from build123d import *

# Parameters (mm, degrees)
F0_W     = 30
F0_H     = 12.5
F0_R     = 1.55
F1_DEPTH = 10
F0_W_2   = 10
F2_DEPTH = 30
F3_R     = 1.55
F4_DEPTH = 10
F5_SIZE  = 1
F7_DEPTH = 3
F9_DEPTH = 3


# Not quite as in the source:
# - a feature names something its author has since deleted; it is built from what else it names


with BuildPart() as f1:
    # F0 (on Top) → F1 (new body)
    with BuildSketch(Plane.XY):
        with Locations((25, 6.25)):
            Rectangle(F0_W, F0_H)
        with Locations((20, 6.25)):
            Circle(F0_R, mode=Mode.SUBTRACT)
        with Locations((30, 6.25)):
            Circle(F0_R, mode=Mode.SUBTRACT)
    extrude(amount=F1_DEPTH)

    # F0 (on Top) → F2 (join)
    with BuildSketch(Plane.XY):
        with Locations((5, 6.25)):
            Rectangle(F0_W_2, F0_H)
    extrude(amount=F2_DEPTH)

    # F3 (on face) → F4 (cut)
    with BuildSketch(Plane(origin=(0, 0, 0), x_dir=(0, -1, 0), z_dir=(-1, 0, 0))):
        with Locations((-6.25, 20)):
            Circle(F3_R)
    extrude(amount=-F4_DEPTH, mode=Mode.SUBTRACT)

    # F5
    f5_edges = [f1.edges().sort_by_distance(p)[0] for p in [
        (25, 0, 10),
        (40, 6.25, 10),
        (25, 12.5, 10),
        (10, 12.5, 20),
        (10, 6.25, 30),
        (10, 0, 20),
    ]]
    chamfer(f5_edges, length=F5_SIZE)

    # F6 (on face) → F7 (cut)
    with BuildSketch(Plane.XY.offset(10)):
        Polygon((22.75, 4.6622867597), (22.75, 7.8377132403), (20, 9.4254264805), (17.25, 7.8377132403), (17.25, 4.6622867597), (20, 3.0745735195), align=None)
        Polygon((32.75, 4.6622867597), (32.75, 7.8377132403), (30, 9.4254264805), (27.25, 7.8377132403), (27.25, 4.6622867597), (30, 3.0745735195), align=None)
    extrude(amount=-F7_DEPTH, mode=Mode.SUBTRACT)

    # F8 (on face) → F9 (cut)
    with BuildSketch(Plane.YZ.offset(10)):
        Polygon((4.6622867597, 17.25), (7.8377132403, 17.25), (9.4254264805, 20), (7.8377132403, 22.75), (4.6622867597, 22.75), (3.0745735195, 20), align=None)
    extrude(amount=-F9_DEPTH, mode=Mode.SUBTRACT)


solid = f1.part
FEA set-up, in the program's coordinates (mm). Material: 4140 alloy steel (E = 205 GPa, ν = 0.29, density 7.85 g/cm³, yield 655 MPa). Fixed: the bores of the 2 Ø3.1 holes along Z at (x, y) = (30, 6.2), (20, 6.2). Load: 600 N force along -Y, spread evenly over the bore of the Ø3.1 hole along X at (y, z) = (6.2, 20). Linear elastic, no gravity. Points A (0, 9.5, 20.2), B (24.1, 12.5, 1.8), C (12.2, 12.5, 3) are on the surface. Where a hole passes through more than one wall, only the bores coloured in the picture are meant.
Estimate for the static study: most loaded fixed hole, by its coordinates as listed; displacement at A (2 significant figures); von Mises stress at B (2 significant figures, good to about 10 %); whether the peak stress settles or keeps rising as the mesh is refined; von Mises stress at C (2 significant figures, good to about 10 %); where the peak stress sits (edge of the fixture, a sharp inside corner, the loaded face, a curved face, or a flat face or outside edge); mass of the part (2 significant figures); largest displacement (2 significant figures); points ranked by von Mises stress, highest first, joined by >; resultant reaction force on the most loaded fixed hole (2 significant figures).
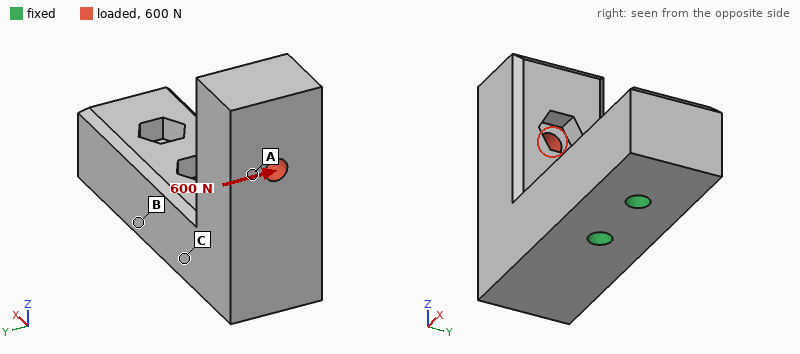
(20, 6.2)
24 µm
23 MPa
keeps rising
48 MPa
edge of the fixture
55 g
34 µm
C > B > A
1.2 kN
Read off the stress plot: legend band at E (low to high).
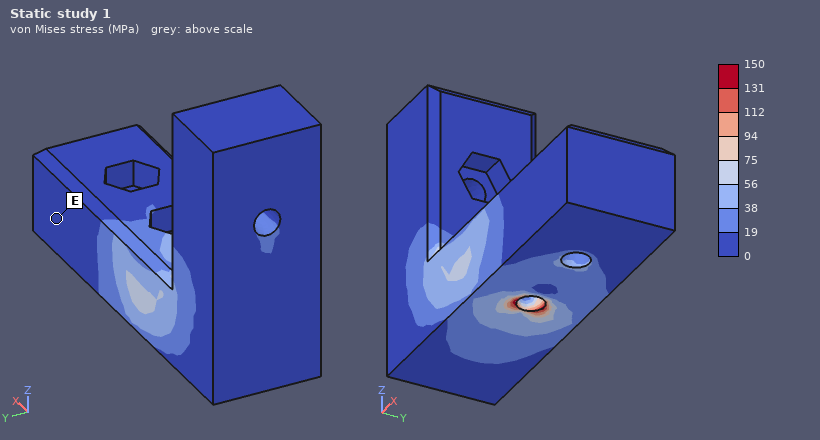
0 to 19 MPa
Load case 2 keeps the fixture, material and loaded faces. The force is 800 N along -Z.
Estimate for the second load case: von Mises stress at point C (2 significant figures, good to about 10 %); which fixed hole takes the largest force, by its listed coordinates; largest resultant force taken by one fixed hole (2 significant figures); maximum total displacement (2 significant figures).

21 MPa
(20, 6.2)
1.3 kN
25 µm
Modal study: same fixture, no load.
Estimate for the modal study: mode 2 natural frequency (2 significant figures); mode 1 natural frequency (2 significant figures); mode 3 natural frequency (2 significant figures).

5800 Hz
5600 Hz
14 kHz
